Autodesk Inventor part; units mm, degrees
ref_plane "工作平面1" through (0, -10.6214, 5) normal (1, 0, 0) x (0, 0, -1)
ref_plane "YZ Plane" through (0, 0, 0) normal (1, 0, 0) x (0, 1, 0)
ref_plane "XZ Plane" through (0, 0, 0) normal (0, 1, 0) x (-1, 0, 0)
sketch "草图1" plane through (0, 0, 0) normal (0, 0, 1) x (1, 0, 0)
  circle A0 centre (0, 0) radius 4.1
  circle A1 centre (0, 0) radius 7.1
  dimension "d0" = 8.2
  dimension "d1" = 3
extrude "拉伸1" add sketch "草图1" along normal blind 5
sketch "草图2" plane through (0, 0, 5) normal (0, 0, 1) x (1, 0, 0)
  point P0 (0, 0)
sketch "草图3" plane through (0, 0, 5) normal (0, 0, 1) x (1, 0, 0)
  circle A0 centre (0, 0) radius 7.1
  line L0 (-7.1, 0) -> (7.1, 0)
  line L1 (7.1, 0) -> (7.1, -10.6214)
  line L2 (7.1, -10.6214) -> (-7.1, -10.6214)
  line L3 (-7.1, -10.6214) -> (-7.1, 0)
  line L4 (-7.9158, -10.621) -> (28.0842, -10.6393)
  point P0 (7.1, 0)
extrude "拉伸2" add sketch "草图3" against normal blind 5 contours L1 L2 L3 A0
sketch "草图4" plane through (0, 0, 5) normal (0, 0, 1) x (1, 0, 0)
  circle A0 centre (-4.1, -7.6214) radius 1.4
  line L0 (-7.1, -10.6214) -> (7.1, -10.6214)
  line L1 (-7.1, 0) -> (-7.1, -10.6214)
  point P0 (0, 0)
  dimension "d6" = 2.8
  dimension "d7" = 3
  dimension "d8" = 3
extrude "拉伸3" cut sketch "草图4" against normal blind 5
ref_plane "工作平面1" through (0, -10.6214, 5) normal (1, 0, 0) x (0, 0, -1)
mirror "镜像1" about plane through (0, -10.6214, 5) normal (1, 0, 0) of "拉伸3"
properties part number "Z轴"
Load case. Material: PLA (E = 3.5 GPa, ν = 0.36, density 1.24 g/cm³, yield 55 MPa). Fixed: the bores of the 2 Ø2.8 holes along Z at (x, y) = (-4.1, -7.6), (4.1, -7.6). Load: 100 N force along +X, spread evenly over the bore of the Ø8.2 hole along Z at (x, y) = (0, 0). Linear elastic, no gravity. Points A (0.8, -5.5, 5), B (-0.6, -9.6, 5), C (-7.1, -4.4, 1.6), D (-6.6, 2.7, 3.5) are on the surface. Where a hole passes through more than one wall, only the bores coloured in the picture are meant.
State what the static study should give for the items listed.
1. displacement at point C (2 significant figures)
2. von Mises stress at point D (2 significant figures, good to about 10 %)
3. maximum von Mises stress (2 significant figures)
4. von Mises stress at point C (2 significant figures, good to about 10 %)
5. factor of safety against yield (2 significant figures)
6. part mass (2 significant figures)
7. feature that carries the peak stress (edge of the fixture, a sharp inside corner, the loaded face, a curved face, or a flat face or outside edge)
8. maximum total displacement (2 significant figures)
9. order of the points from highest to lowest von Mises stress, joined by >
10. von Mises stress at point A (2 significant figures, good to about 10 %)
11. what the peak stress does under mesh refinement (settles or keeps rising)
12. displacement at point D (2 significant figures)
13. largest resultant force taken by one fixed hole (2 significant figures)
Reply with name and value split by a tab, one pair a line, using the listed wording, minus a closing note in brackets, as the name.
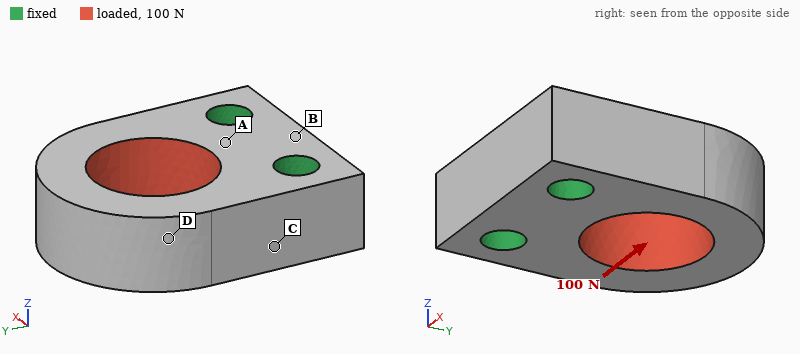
displacement at point C	11 µm
von Mises stress at point D	3.2 MPa
maximum von Mises stress	11 MPa
von Mises stress at point C	7.5 MPa
factor of safety against yield	4.9
part mass	1.0 g
feature that carries the peak stress	the loaded face
maximum total displacement	55 µm
order of the points from highest to lowest von Mises stress, joined by >	C > A > D > B
von Mises stress at point A	5.6 MPa
what the peak stress does under mesh refinement	settles
displacement at point D	48 µm
largest resultant force taken by one fixed hole	76 N
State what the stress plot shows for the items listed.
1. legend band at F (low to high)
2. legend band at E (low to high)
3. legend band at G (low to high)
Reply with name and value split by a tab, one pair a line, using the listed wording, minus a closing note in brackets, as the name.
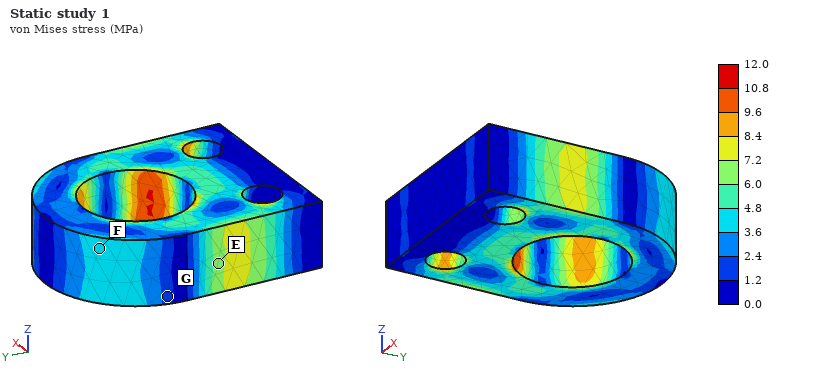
legend band at F	3.6 to 4.8 MPa
legend band at E	6.0 to 7.2 MPa
legend band at G	1.2 to 2.4 MPa
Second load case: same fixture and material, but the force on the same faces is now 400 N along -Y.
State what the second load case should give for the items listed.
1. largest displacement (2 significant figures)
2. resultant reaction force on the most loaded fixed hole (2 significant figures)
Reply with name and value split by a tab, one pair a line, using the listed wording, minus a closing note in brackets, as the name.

largest displacement	50 µm
resultant reaction force on the most loaded fixed hole	200 N
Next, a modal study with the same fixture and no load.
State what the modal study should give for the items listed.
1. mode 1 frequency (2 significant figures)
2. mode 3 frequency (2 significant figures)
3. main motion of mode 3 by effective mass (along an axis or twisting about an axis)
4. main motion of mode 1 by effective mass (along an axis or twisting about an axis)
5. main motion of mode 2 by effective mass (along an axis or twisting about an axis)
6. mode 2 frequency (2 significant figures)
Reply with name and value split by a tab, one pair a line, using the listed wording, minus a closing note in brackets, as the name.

mode 1 frequency	6600 Hz
mode 3 frequency	14 kHz
main motion of mode 3 by effective mass	twisting about Y
main motion of mode 1 by effective mass	along Z
main motion of mode 2 by effective mass	along X
mode 2 frequency	9200 Hz
